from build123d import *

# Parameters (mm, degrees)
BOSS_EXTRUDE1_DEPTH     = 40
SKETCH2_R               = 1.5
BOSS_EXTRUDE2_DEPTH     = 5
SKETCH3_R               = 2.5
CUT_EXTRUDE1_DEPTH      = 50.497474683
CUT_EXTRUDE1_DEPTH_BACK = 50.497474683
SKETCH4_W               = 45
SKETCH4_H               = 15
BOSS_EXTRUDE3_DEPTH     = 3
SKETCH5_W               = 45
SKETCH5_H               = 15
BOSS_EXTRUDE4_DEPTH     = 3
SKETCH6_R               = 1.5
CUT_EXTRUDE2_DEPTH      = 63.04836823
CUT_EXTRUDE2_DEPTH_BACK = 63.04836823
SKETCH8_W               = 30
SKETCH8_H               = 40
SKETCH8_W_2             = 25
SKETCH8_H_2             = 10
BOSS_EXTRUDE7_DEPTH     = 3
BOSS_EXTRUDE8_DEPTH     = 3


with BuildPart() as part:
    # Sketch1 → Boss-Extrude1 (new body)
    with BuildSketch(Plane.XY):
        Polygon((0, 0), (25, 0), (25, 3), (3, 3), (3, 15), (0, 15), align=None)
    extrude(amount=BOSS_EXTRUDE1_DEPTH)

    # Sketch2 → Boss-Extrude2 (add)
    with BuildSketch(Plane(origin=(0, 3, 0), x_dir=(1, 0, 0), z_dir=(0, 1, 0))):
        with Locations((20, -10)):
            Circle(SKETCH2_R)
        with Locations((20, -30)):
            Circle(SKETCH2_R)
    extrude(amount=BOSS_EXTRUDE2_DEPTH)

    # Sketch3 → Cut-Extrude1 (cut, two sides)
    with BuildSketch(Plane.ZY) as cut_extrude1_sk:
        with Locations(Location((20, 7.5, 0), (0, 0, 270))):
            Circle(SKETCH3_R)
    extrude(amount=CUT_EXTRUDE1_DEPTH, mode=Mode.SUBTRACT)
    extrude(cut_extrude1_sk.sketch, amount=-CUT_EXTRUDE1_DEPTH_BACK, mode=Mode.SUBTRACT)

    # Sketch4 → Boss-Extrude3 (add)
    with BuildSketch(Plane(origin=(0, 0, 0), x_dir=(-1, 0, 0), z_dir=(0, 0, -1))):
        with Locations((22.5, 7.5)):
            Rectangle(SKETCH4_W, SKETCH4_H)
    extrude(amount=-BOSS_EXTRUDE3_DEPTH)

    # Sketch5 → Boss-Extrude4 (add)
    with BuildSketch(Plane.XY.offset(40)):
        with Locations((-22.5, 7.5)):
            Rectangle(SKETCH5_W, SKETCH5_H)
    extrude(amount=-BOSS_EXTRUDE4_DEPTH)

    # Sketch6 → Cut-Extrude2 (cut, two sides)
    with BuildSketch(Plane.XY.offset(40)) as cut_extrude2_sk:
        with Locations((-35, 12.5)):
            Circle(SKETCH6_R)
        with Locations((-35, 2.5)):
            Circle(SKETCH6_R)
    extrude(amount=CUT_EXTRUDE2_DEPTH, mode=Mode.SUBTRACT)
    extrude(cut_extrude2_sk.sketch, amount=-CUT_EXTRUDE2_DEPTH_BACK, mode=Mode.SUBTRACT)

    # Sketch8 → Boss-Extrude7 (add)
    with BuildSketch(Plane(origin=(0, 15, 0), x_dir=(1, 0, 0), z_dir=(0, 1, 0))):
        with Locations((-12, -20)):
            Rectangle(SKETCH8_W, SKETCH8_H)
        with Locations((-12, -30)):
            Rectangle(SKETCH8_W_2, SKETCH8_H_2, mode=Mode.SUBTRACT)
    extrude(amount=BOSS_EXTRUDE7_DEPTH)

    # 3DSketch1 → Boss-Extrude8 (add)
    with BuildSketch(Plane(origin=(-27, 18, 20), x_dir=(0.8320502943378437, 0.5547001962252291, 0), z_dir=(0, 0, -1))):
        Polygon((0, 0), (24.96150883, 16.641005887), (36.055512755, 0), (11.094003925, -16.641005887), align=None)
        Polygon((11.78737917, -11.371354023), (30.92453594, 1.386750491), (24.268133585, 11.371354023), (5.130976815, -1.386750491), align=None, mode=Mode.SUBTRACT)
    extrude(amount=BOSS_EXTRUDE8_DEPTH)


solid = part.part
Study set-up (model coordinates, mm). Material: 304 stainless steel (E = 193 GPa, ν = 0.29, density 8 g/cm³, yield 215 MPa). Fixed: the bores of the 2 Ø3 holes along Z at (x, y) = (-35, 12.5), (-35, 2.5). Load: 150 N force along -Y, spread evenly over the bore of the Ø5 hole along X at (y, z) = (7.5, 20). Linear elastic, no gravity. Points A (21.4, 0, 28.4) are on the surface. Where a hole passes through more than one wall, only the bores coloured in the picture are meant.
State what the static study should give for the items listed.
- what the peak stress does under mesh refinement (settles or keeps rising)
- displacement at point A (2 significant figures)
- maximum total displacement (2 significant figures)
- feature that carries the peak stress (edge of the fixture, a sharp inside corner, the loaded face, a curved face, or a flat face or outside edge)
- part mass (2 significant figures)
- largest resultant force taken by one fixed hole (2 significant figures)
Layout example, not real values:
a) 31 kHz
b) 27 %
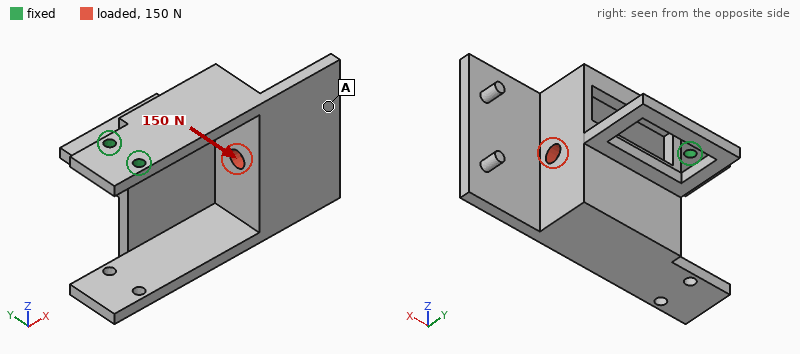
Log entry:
a) keeps rising
b) 0.088 mm
c) 0.27 mm
d) edge of the fixture
e) 98 g
f) 550 N
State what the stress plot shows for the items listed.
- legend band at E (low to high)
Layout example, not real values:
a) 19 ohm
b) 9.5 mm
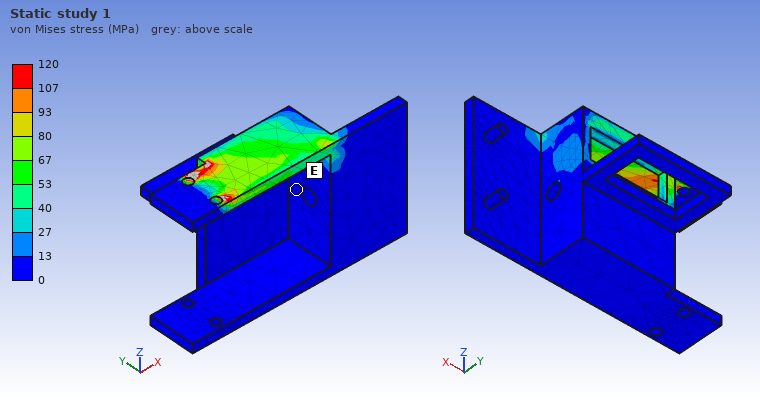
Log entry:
a) 0 to 13 MPa
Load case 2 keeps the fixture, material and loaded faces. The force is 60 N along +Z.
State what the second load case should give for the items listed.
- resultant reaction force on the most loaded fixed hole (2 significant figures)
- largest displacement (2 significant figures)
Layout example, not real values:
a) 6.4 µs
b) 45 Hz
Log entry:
a) 30 N
b) 0.25 mm
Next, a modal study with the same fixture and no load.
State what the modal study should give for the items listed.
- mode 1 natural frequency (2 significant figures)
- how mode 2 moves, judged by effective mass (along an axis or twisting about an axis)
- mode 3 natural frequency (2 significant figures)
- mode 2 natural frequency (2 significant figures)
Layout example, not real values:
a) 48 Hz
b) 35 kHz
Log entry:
a) 310 Hz
b) along Y
c) 1300 Hz
d) 440 Hz
